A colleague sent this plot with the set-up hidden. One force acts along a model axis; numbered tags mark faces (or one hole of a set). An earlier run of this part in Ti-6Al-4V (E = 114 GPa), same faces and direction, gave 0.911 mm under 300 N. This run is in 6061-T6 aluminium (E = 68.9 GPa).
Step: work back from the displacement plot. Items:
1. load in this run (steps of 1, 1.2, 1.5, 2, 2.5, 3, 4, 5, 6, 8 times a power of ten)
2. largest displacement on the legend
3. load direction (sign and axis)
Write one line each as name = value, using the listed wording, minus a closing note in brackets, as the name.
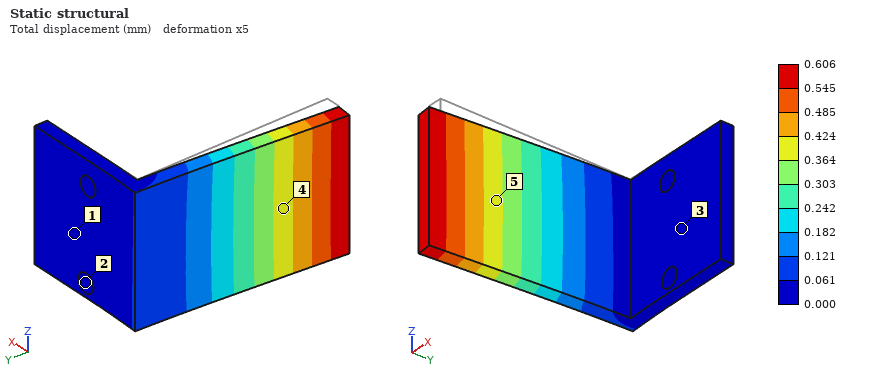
load in this run = 120 N
largest displacement on the legend = 0.606 mm
load direction = -X
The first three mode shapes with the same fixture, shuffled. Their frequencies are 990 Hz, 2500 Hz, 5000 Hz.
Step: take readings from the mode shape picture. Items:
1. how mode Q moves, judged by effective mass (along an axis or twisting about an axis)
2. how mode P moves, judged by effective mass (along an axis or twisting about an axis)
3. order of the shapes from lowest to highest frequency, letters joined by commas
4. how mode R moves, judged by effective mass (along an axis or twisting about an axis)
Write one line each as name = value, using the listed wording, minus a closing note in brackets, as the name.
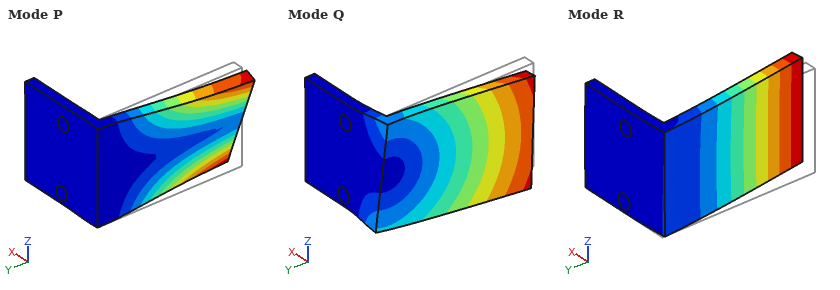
how mode Q moves, judged by effective mass = along Z
how mode P moves, judged by effective mass = twisting about Y
order of the shapes from lowest to highest frequency, letters joined by commas = R, Q, P
how mode R moves, judged by effective mass = along X
